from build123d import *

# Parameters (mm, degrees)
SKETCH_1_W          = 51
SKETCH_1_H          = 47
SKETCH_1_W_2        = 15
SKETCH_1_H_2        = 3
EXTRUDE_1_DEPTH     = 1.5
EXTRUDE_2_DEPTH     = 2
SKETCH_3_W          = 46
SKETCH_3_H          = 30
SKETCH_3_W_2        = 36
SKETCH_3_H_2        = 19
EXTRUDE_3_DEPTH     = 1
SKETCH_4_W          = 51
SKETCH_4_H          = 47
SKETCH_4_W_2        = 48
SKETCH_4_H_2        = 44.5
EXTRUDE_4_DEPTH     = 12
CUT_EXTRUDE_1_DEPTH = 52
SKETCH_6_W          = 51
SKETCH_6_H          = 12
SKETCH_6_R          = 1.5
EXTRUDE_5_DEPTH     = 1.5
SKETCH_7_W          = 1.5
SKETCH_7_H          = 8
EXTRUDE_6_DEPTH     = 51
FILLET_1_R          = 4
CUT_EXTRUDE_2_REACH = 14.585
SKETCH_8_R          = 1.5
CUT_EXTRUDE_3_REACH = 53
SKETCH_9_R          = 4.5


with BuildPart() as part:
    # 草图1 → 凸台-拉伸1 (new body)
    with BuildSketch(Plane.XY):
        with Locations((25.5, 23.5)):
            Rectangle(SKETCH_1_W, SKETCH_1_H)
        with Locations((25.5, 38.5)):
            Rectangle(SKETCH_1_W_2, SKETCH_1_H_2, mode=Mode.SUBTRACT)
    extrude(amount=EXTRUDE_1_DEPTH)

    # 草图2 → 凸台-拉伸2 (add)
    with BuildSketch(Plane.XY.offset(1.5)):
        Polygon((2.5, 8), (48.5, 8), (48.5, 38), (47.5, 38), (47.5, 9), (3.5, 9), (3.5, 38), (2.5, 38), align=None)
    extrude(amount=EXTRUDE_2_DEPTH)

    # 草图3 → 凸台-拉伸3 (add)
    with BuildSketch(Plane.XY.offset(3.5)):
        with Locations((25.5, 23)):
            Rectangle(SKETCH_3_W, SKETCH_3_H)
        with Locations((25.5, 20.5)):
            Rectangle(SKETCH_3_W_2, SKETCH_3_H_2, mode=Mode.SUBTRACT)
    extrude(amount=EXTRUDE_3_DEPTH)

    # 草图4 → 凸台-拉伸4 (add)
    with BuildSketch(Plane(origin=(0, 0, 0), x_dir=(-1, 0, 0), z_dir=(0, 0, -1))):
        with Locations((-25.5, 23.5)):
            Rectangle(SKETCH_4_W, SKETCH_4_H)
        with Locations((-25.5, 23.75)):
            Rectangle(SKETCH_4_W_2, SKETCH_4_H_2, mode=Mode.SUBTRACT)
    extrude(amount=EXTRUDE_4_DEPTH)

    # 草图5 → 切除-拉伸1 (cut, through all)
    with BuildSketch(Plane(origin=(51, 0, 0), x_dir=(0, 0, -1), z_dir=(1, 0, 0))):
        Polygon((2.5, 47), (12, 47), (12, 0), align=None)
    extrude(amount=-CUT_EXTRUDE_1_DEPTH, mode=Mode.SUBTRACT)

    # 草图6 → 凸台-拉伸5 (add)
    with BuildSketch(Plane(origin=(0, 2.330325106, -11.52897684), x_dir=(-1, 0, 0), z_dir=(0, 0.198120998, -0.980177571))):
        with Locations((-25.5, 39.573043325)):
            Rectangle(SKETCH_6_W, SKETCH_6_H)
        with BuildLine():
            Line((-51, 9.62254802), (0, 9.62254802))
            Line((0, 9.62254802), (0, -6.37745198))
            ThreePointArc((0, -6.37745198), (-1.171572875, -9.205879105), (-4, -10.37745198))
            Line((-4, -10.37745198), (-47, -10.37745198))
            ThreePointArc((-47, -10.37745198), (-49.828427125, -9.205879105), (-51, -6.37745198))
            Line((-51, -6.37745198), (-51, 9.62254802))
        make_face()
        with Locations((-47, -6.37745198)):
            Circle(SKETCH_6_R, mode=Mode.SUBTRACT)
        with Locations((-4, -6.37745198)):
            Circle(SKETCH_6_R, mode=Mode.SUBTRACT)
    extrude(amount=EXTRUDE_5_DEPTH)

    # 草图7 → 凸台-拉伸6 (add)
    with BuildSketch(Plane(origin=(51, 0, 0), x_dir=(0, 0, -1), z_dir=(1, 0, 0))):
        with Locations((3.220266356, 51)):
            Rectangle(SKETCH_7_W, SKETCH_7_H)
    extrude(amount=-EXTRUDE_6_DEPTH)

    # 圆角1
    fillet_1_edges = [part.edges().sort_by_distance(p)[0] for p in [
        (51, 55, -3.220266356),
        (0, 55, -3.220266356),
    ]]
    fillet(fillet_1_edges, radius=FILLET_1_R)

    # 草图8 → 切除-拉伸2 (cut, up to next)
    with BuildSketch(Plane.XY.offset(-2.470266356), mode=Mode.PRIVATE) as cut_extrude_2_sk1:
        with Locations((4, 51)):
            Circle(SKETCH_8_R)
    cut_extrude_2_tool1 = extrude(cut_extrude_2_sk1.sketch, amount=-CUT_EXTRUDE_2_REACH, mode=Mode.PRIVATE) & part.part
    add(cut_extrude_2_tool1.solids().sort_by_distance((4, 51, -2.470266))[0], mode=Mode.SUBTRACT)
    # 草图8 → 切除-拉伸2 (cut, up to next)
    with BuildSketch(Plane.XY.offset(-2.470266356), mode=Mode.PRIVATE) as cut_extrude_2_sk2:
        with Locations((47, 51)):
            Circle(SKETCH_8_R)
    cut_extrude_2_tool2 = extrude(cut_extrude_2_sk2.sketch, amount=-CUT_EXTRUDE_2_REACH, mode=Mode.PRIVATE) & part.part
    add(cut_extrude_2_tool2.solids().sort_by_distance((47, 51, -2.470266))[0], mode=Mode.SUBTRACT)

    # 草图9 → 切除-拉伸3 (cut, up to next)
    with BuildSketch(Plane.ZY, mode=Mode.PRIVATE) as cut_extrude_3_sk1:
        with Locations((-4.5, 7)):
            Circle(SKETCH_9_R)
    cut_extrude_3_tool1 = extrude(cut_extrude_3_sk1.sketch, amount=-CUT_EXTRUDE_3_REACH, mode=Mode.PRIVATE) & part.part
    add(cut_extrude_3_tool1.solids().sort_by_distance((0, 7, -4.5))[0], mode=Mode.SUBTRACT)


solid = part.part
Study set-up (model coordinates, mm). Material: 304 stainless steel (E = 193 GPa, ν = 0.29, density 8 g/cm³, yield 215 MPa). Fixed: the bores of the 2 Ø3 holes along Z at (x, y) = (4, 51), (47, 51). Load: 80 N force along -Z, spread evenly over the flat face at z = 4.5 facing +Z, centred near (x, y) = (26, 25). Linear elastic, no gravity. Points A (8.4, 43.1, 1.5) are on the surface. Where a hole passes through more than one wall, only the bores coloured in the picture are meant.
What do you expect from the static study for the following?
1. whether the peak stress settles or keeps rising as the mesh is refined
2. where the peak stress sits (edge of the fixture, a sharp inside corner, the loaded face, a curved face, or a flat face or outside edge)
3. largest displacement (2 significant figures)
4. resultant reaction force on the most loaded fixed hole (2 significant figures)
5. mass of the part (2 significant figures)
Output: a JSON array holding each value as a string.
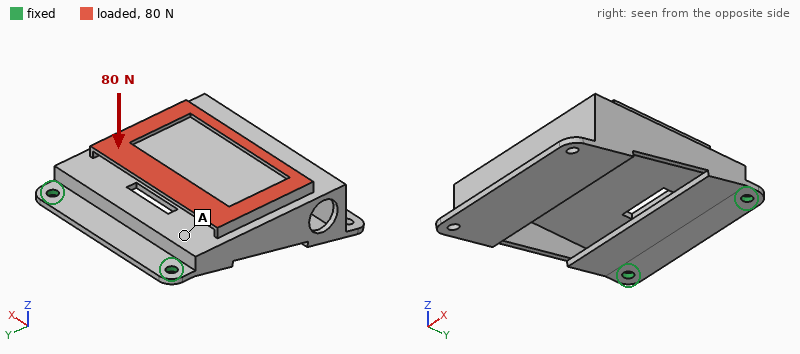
["keeps rising", "edge of the fixture", "0.34 mm", "60 N", "75 g"]
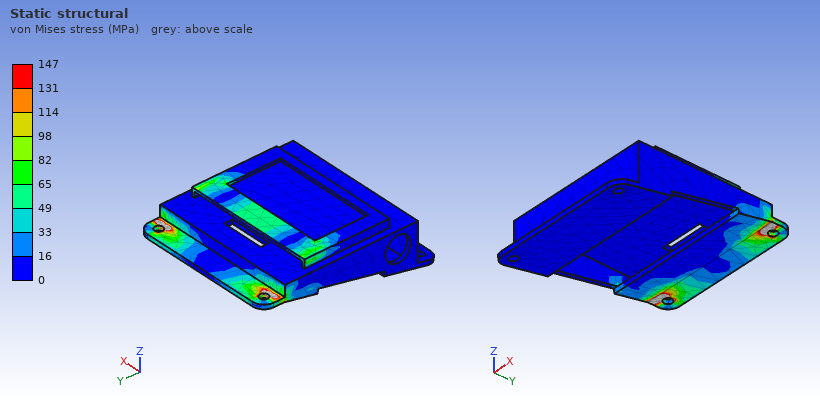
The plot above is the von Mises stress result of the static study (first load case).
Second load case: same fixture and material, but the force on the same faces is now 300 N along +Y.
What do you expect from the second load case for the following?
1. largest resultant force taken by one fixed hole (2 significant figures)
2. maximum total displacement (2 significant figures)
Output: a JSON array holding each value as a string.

["160 N", "0.42 mm"]
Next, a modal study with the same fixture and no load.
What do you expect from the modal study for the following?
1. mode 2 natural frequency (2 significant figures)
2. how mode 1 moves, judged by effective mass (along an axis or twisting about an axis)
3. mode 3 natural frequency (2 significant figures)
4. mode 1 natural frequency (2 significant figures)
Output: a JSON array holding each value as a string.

["1000 Hz", "along Z", "2500 Hz", "310 Hz"]
